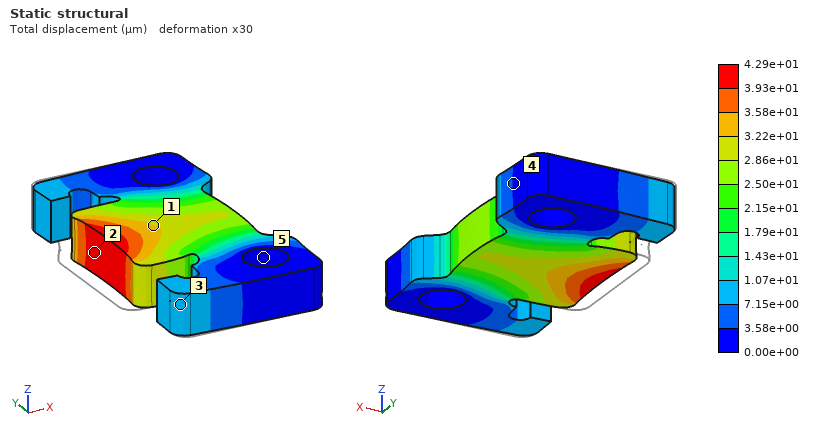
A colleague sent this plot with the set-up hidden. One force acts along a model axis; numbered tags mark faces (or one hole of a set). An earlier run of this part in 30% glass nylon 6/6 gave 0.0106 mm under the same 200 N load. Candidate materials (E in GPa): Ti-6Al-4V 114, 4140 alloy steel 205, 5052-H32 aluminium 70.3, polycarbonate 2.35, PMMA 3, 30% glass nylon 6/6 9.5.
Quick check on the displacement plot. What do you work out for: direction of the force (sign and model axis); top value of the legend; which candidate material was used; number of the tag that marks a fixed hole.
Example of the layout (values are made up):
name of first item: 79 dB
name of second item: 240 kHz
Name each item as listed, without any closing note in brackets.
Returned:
direction of the force: +X
top value of the legend: 4.29e+01 µm
which candidate material was used: polycarbonate
number of the tag that marks a fixed hole: 5
